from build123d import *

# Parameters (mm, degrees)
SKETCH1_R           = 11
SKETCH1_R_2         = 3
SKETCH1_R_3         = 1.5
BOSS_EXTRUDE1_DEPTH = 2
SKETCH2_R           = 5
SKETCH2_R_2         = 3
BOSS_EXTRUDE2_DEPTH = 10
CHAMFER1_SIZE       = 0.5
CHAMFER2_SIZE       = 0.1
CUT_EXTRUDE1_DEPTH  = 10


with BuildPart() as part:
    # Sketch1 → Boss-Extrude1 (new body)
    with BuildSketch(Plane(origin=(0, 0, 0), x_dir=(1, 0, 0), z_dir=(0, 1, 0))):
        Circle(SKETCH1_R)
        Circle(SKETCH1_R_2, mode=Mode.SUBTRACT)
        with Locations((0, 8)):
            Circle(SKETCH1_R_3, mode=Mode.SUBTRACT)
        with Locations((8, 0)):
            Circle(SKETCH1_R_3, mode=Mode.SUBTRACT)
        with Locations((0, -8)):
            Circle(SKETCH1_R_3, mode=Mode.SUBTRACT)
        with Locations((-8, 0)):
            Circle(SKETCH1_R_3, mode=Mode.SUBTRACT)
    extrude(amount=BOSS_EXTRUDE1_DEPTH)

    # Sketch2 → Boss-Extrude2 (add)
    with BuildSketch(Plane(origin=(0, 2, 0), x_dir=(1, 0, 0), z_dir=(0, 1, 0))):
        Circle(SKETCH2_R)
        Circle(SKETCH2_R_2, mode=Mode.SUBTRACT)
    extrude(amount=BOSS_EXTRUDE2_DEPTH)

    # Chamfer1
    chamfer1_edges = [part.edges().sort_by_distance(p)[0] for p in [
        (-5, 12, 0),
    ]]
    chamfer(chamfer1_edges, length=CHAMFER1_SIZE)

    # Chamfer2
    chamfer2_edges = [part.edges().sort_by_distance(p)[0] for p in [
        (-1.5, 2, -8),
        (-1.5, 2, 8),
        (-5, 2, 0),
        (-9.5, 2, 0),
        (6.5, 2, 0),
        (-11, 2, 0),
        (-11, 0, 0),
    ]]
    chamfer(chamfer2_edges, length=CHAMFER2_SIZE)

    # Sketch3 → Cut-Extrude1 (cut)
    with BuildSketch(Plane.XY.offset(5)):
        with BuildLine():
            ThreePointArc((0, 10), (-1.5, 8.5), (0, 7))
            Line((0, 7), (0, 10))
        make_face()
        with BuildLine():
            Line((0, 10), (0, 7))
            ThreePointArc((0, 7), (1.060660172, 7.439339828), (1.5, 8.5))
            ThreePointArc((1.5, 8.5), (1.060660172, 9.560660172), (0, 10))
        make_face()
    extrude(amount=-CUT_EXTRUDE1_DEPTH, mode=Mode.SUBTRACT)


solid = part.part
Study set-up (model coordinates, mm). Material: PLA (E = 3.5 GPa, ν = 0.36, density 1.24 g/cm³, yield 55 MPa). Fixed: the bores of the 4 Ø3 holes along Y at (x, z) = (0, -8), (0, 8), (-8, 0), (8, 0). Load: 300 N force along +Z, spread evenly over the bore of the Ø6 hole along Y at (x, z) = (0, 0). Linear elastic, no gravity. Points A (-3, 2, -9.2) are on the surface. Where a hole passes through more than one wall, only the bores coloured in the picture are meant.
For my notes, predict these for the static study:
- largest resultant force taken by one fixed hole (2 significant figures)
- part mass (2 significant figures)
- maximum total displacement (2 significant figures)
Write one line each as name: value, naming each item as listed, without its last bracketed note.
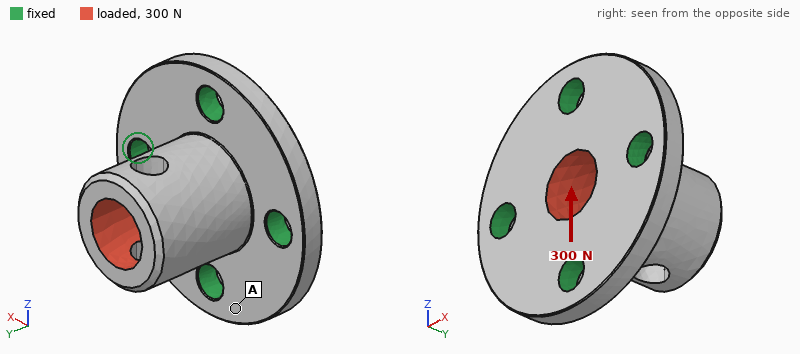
largest resultant force taken by one fixed hole: 150 N
part mass: 1.4 g
maximum total displacement: 0.13 mm
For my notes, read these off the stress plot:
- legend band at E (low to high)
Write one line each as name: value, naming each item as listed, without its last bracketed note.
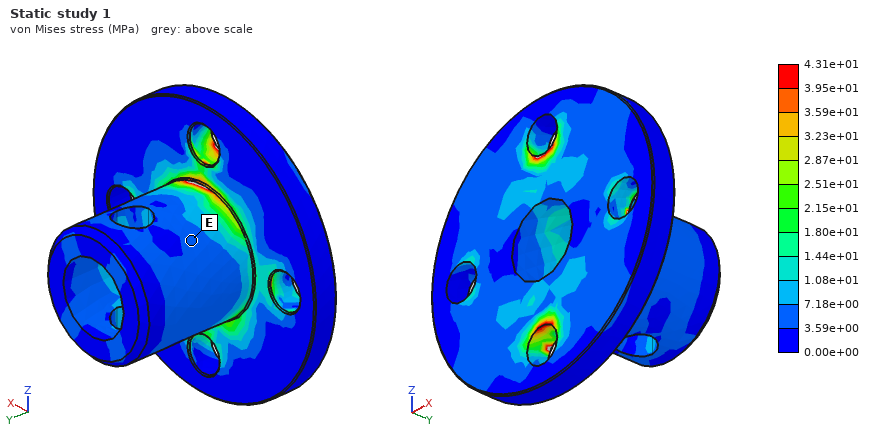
legend band at E: 3.59e+00 to 7.18e+00 MPa
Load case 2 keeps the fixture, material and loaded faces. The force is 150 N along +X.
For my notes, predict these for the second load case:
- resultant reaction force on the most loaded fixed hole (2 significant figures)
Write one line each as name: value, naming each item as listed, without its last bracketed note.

resultant reaction force on the most loaded fixed hole: 74 N
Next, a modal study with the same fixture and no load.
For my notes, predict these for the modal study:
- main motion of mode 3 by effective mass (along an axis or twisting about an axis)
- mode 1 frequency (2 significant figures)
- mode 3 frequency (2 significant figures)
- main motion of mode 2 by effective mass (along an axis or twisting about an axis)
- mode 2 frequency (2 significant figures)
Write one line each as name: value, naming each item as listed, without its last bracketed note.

main motion of mode 3 by effective mass: along Y
mode 1 frequency: 10 kHz
mode 3 frequency: 18 kHz
main motion of mode 2 by effective mass: along Z
mode 2 frequency: 11 kHz
